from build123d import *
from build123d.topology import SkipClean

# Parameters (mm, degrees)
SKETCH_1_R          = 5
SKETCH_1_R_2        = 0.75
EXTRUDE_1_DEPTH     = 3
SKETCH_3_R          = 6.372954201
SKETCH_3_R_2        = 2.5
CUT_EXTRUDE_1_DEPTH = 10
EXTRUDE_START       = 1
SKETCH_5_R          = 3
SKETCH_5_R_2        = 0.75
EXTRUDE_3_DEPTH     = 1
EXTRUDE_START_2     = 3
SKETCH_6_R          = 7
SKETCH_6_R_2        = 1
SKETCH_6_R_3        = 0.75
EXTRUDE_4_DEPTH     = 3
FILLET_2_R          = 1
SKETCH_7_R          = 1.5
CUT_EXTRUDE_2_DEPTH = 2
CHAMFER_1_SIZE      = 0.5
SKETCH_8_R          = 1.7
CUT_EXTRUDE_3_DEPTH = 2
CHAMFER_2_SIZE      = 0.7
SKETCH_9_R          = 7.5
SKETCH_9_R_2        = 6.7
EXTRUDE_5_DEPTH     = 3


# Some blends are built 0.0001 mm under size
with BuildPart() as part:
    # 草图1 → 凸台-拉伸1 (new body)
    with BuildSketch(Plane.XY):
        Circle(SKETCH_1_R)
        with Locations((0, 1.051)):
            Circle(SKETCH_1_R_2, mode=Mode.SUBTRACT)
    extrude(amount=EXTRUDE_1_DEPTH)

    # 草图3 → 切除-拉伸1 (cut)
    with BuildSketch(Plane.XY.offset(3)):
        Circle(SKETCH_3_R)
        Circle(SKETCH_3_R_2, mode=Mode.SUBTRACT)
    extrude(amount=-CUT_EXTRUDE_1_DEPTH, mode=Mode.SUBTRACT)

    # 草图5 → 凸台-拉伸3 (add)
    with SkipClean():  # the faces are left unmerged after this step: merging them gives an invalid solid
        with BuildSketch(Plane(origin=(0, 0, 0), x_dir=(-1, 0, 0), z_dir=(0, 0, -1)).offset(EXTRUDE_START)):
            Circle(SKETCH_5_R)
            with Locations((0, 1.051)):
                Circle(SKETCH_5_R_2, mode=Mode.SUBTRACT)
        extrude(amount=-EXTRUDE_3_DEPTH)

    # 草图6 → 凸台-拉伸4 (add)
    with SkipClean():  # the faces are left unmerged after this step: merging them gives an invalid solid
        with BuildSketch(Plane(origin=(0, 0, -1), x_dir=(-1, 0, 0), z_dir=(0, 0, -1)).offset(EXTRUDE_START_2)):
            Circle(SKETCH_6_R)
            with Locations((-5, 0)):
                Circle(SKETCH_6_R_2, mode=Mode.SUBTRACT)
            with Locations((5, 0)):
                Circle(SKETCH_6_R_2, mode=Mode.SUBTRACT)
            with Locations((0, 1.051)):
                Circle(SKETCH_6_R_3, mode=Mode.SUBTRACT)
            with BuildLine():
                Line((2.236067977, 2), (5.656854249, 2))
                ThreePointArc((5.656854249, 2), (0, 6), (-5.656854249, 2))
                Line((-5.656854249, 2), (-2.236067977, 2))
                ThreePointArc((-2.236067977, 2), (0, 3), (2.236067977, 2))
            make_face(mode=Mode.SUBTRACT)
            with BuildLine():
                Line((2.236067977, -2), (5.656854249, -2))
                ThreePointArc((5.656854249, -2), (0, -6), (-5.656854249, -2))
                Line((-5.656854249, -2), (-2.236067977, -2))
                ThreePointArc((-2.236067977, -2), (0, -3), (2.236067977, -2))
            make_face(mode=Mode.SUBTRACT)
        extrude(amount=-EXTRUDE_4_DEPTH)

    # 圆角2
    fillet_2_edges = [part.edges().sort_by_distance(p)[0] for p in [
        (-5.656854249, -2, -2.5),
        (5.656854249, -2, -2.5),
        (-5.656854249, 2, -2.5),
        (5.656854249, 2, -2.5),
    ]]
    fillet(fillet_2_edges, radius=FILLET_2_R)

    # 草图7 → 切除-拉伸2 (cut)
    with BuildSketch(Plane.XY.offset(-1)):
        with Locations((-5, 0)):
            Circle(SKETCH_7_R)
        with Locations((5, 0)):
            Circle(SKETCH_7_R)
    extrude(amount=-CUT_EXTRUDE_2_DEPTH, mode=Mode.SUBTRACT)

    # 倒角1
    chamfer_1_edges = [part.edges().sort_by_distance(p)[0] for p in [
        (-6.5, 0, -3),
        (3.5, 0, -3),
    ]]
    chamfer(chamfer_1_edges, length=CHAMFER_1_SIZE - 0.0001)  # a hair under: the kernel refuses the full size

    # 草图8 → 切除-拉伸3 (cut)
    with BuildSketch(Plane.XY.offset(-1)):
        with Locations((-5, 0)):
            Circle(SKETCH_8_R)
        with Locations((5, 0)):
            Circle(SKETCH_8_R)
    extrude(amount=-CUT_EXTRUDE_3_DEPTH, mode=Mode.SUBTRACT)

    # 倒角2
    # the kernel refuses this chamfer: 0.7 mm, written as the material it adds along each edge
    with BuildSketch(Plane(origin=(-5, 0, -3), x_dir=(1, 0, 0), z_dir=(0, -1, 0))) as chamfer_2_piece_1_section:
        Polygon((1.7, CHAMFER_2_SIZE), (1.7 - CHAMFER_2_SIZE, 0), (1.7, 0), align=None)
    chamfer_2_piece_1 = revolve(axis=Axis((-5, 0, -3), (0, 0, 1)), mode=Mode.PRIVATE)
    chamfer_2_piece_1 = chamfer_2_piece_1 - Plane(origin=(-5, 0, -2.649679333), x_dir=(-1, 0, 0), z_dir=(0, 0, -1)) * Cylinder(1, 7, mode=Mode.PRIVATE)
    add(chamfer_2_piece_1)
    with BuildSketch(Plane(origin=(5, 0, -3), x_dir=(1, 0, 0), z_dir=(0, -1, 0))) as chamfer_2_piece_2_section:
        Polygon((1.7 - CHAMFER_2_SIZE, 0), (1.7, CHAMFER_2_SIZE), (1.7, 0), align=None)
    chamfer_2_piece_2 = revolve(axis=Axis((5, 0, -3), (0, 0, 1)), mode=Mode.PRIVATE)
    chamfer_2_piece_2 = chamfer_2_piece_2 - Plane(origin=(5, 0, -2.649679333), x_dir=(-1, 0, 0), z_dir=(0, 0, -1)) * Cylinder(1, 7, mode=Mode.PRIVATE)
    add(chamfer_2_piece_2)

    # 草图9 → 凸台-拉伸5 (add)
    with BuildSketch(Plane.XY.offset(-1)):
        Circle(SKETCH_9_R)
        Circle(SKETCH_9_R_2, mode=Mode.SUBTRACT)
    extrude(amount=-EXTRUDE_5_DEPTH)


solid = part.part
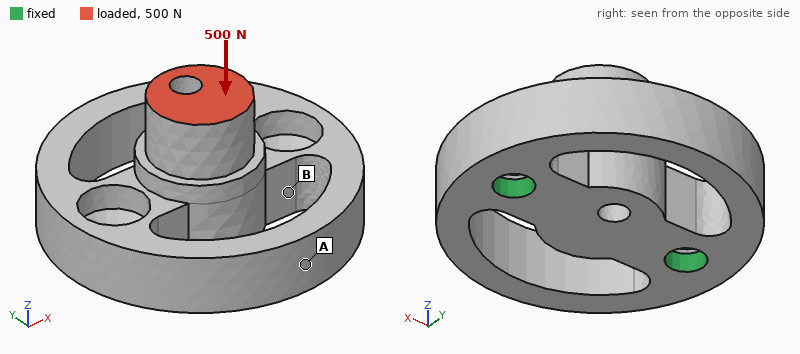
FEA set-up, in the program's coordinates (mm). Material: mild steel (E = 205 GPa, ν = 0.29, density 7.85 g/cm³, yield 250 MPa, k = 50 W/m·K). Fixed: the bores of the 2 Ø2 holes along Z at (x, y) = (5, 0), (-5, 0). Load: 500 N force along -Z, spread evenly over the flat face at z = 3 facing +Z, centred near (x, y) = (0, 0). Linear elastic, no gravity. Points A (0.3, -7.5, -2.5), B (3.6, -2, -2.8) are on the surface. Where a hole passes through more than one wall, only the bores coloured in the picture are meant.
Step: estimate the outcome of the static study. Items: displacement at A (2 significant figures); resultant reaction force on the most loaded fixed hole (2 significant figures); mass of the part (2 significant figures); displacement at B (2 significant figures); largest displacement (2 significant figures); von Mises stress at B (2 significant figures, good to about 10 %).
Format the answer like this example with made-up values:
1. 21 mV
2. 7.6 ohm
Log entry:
1. 1.1 µm
2. 300 N
3. 3.1 g
4. 1.0 µm
5. 2.5 µm
6. 42 MPa
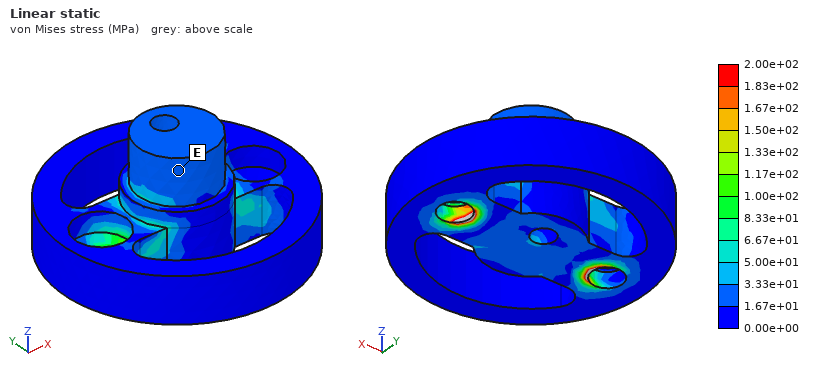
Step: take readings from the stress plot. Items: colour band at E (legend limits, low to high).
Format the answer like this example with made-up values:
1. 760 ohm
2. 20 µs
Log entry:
1. 1.67e+01 to 3.33e+01 MPa
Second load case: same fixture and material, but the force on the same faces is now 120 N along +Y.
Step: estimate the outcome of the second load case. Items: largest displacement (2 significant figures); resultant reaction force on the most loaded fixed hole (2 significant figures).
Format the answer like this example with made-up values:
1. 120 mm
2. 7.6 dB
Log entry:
1. 9.7 µm
2. 60 N
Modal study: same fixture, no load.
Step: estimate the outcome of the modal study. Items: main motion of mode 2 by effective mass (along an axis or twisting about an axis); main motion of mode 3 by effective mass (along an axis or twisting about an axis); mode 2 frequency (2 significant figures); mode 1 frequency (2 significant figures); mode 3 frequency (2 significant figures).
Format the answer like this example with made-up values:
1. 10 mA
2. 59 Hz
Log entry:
1. along Z
2. along Y
3. 28 kHz
4. 21 kHz
5. 35 kHz
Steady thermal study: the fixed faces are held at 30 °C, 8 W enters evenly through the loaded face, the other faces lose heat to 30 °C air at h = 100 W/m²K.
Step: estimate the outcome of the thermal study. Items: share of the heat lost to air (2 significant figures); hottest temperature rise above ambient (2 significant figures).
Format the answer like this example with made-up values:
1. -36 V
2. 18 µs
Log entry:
1. 10 %
2. 63 K
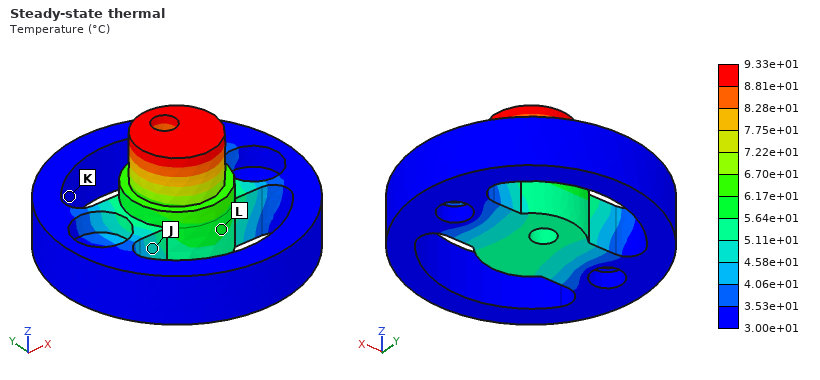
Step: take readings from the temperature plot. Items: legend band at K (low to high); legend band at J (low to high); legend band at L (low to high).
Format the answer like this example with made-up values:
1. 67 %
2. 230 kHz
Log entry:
1. 3.00e+01 to 3.53e+01 °C
2. 4.58e+01 to 5.11e+01 °C
3. 5.64e+01 to 6.17e+01 °C
